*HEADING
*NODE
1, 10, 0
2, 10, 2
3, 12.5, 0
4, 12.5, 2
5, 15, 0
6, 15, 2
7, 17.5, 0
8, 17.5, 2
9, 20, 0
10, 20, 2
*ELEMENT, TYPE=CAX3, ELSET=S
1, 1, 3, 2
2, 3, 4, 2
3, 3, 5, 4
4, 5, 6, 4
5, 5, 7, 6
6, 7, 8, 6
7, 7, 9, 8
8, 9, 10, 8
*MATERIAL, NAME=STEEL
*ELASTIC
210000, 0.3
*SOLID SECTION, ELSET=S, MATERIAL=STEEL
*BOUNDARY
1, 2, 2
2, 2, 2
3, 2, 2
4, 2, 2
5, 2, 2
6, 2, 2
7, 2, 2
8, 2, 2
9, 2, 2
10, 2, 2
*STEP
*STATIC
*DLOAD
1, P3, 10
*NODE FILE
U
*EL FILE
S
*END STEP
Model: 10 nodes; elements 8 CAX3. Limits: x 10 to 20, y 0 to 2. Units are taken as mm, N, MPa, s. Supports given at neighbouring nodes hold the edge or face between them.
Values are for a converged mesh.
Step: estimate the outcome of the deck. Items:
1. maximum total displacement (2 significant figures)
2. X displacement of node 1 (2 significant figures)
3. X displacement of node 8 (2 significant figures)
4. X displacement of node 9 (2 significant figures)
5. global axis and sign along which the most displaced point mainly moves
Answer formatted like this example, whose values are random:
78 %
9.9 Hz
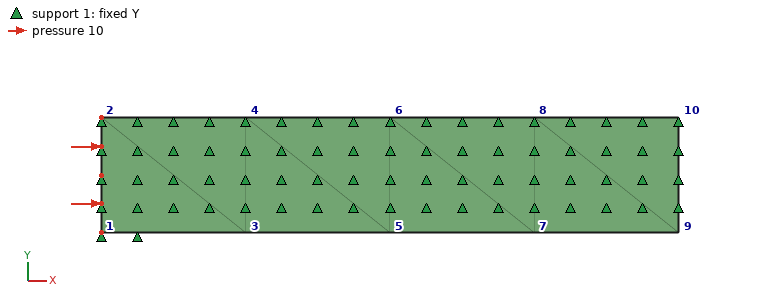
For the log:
9.1e-04 mm
9.1e-04 mm
6.2e-04 mm
5.8e-04 mm
+X
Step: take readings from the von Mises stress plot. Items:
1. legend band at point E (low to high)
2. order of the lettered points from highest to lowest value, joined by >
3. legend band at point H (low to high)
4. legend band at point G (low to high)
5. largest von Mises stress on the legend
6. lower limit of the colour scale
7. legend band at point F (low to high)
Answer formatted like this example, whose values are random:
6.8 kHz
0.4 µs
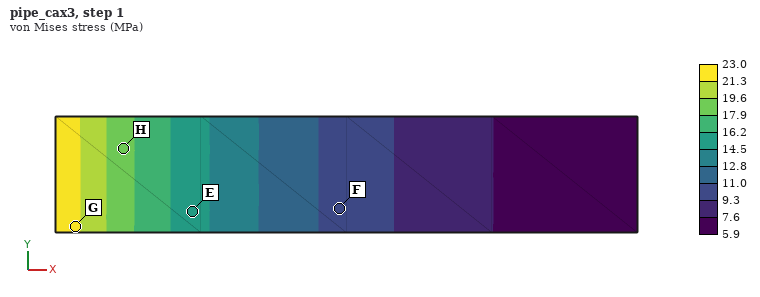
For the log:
14.5 to 16.2 MPa
G > H > E > F
17.9 to 19.6 MPa
21.3 to 23.0 MPa
23.0 MPa
5.9 MPa
9.3 to 11.0 MPa
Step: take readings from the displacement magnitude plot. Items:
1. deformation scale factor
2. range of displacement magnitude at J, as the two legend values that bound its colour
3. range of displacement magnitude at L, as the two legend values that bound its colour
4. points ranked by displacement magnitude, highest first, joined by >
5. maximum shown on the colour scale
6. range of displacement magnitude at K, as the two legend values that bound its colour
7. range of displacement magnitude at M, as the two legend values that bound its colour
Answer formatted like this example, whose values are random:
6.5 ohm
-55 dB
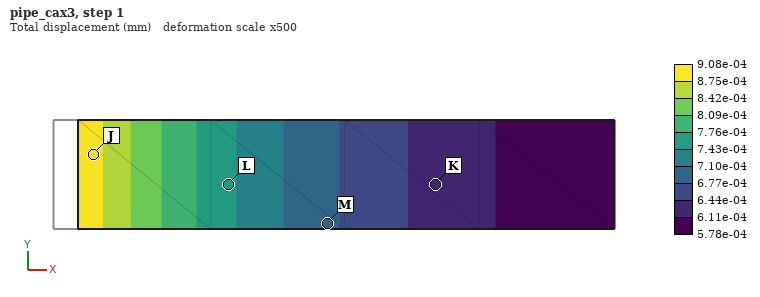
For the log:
500
8.75e-04 to 9.08e-04 mm
7.43e-04 to 7.76e-04 mm
J > L > M > K
9.08e-04 mm
6.11e-04 to 6.44e-04 mm
6.77e-04 to 7.10e-04 mm
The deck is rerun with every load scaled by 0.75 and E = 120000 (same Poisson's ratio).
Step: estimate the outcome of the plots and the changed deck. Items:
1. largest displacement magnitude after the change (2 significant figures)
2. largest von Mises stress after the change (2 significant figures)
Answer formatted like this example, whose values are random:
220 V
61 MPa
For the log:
0.0012 mm
17 MPa
